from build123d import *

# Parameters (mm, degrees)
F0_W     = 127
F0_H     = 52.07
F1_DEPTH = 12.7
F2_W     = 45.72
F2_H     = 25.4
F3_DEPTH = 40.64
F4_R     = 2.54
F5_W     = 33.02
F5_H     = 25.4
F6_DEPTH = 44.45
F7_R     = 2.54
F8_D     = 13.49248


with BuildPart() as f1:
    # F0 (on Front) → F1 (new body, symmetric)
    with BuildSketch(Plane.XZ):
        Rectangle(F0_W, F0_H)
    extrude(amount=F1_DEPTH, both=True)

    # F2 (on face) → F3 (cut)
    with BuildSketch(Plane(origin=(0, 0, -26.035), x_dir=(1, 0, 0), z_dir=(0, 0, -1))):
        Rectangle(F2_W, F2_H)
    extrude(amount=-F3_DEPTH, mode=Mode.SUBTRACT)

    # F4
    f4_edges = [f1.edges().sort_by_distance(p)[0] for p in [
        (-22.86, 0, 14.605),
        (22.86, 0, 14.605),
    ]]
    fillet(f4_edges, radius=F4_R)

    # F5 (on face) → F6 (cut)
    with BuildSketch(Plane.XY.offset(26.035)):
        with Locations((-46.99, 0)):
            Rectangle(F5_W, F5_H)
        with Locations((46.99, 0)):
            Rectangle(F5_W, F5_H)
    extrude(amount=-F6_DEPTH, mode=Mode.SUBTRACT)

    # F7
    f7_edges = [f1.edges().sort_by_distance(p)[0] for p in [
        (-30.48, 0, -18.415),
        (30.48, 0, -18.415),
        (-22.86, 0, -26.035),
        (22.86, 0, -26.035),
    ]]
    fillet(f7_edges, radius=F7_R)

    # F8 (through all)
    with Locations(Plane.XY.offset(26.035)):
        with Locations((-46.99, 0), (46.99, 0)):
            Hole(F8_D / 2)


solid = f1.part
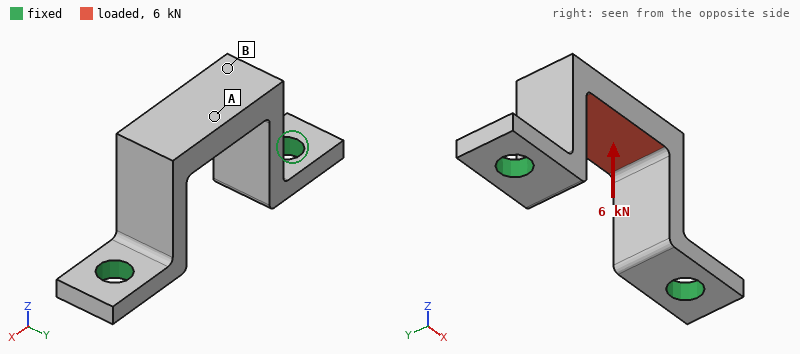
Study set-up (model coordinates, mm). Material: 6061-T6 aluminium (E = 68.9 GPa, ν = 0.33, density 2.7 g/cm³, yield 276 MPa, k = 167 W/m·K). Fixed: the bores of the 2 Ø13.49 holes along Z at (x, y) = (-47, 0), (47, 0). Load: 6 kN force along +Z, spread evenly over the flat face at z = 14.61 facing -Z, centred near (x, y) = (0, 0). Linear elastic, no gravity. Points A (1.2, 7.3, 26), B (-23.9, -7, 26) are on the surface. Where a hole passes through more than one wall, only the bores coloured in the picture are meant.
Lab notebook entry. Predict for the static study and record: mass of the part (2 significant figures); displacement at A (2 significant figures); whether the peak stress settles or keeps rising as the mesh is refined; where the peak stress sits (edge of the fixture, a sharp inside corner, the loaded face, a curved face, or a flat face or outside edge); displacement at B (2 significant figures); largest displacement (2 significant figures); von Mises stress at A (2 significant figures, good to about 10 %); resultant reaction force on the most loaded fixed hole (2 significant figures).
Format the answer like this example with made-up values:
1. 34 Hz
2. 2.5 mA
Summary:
1. 120 g
2. 71 µm
3. keeps rising
4. edge of the fixture
5. 42 µm
6. 74 µm
7. 53 MPa
8. 3.2 kN
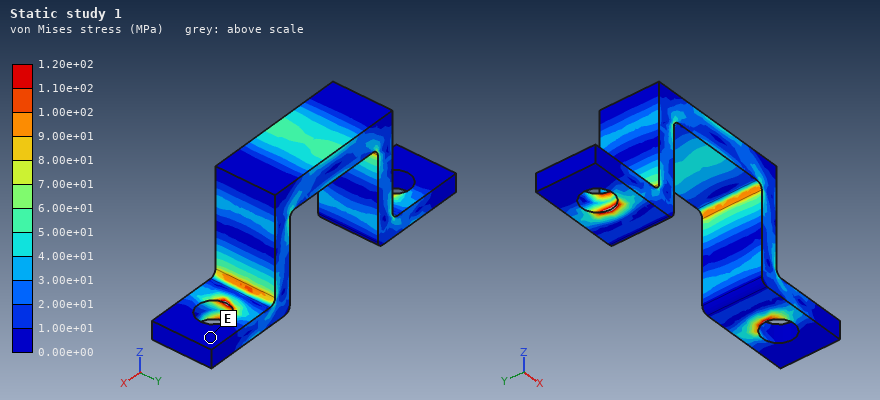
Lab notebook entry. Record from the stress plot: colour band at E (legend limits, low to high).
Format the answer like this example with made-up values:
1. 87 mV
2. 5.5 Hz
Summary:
1. 0.00e+00 to 1.00e+01 MPa
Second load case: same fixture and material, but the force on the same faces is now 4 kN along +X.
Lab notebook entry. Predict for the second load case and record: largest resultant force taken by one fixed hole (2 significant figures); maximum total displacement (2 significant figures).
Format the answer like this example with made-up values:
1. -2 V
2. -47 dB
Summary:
1. 2.5 kN
2. 0.24 mm
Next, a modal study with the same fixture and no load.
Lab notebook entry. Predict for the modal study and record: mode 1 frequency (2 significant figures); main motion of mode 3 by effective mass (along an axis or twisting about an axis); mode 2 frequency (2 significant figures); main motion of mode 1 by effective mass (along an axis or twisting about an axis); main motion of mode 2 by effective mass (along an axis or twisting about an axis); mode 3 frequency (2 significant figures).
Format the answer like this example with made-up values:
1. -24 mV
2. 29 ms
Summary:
1. 1800 Hz
2. twisting about Z
3. 2700 Hz
4. along Y
5. along X
6. 4000 Hz
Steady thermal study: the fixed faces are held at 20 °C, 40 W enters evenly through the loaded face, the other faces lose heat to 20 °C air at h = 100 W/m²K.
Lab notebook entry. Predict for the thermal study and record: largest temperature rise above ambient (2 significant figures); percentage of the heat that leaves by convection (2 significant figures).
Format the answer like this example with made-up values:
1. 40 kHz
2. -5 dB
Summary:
1. 28 K
2. 38 %
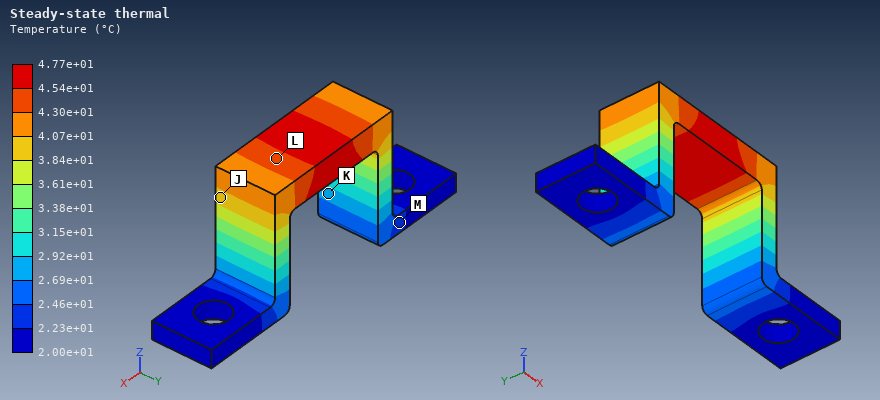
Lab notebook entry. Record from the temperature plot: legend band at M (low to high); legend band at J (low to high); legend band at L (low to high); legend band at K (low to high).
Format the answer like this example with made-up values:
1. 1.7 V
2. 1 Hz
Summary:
1. 2.23e+01 to 2.46e+01 °C
2. 3.84e+01 to 4.07e+01 °C
3. 4.30e+01 to 4.54e+01 °C
4. 2.69e+01 to 2.92e+01 °C
